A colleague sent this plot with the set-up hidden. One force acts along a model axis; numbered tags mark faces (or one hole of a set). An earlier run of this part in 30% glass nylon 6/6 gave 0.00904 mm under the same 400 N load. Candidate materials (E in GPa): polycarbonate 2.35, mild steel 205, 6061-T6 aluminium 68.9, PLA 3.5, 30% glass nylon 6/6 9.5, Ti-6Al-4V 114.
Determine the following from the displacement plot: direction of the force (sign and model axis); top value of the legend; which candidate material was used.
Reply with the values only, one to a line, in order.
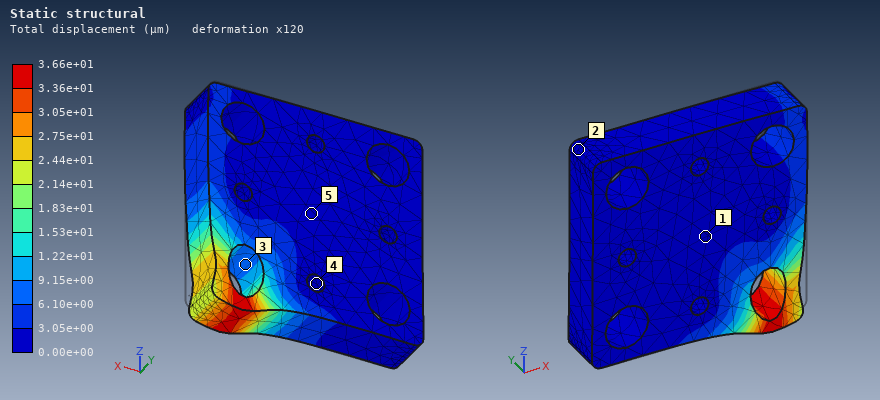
-Z
3.66e+01 µm
polycarbonate
